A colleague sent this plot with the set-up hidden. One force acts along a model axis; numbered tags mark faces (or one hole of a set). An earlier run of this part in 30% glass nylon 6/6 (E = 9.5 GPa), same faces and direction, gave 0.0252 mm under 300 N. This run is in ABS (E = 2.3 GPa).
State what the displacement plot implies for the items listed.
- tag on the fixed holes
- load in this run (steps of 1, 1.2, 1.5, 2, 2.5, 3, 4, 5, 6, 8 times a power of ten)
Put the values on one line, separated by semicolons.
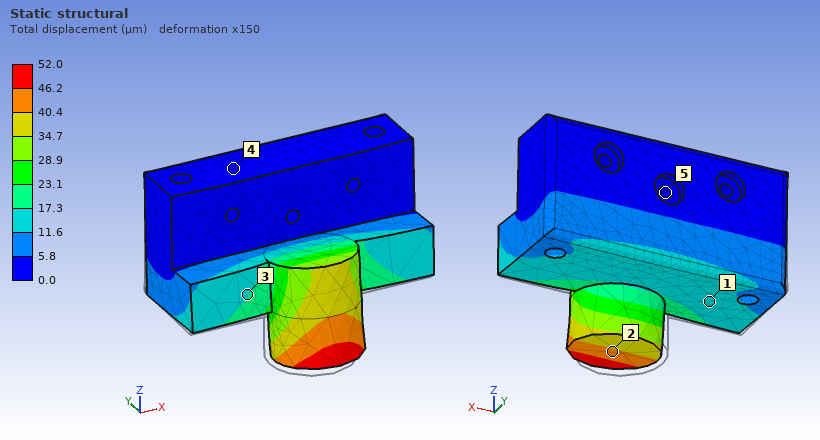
5; 150 N
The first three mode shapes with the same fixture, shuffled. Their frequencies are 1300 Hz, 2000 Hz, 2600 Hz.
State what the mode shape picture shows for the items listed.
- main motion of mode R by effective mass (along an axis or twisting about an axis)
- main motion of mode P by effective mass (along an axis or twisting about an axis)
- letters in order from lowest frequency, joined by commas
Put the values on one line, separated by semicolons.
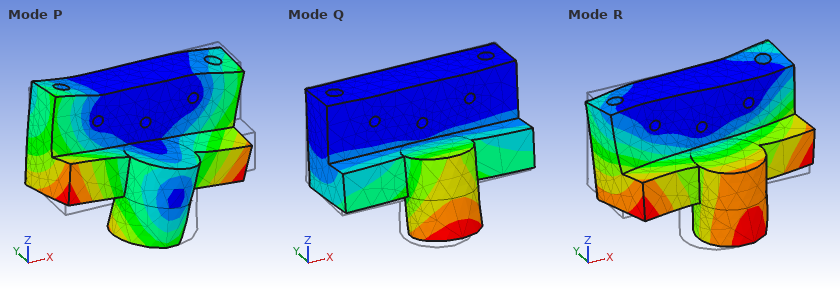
along X; along X; Q, R, P
